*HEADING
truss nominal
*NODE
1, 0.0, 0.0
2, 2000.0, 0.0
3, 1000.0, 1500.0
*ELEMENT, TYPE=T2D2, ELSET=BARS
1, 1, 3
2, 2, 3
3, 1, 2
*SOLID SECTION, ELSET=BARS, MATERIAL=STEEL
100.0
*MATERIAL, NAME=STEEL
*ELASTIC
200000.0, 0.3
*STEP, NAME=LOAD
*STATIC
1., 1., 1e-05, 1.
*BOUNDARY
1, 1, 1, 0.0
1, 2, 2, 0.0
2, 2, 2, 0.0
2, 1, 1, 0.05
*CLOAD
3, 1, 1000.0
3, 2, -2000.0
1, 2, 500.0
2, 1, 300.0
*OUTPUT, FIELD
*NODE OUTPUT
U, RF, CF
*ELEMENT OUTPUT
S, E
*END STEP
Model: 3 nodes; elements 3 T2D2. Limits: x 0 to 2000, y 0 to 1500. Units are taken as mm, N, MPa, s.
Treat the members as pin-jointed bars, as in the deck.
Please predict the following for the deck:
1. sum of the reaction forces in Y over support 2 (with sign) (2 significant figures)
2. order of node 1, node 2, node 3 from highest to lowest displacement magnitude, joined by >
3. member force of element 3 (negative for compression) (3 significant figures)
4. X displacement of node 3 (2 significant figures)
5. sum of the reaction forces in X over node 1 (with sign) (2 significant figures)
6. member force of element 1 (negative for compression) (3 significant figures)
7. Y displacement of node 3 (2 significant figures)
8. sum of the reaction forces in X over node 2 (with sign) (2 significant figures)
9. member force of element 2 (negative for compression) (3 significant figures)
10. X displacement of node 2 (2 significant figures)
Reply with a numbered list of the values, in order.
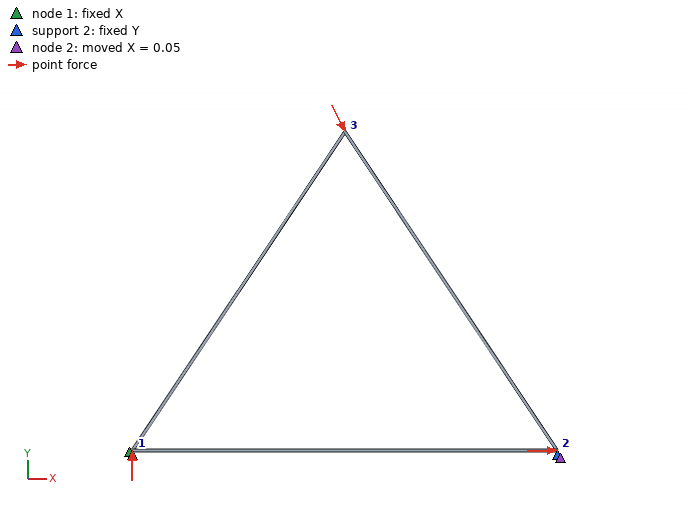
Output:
1. 1500 N
2. node 3 > node 2 > node 1
3. 500 N
4. 0.17 mm
5. -330 N
6. -300 N
7. -0.15 mm
8. -970 N
9. -2100 N
10. 0.050 mm
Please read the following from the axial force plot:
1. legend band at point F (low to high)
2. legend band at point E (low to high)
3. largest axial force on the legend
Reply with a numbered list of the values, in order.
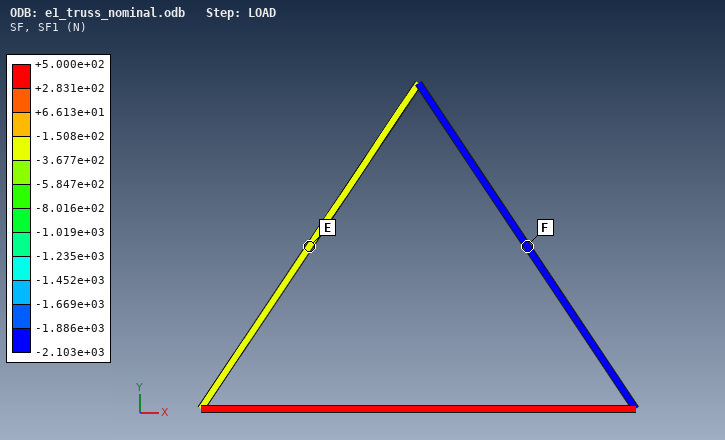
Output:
1. -2.103e+03 to -1.886e+03 N
2. -3.677e+02 to -1.508e+02 N
3. +5.000e+02 N
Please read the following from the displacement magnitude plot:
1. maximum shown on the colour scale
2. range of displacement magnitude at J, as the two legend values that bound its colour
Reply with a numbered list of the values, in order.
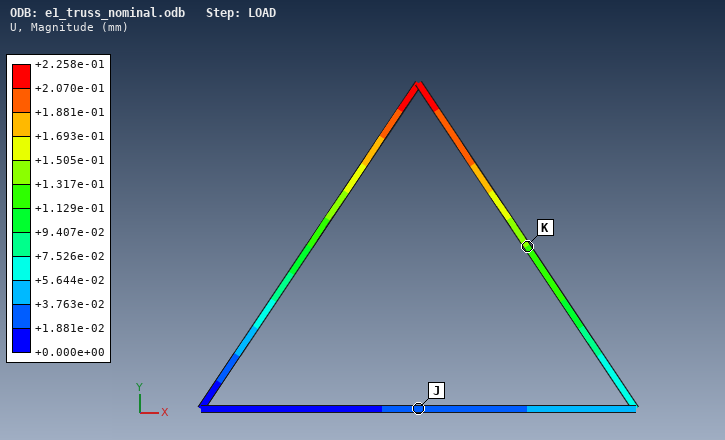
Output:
1. +2.258e-01 mm
2. +1.881e-02 to +3.763e-02 mm
